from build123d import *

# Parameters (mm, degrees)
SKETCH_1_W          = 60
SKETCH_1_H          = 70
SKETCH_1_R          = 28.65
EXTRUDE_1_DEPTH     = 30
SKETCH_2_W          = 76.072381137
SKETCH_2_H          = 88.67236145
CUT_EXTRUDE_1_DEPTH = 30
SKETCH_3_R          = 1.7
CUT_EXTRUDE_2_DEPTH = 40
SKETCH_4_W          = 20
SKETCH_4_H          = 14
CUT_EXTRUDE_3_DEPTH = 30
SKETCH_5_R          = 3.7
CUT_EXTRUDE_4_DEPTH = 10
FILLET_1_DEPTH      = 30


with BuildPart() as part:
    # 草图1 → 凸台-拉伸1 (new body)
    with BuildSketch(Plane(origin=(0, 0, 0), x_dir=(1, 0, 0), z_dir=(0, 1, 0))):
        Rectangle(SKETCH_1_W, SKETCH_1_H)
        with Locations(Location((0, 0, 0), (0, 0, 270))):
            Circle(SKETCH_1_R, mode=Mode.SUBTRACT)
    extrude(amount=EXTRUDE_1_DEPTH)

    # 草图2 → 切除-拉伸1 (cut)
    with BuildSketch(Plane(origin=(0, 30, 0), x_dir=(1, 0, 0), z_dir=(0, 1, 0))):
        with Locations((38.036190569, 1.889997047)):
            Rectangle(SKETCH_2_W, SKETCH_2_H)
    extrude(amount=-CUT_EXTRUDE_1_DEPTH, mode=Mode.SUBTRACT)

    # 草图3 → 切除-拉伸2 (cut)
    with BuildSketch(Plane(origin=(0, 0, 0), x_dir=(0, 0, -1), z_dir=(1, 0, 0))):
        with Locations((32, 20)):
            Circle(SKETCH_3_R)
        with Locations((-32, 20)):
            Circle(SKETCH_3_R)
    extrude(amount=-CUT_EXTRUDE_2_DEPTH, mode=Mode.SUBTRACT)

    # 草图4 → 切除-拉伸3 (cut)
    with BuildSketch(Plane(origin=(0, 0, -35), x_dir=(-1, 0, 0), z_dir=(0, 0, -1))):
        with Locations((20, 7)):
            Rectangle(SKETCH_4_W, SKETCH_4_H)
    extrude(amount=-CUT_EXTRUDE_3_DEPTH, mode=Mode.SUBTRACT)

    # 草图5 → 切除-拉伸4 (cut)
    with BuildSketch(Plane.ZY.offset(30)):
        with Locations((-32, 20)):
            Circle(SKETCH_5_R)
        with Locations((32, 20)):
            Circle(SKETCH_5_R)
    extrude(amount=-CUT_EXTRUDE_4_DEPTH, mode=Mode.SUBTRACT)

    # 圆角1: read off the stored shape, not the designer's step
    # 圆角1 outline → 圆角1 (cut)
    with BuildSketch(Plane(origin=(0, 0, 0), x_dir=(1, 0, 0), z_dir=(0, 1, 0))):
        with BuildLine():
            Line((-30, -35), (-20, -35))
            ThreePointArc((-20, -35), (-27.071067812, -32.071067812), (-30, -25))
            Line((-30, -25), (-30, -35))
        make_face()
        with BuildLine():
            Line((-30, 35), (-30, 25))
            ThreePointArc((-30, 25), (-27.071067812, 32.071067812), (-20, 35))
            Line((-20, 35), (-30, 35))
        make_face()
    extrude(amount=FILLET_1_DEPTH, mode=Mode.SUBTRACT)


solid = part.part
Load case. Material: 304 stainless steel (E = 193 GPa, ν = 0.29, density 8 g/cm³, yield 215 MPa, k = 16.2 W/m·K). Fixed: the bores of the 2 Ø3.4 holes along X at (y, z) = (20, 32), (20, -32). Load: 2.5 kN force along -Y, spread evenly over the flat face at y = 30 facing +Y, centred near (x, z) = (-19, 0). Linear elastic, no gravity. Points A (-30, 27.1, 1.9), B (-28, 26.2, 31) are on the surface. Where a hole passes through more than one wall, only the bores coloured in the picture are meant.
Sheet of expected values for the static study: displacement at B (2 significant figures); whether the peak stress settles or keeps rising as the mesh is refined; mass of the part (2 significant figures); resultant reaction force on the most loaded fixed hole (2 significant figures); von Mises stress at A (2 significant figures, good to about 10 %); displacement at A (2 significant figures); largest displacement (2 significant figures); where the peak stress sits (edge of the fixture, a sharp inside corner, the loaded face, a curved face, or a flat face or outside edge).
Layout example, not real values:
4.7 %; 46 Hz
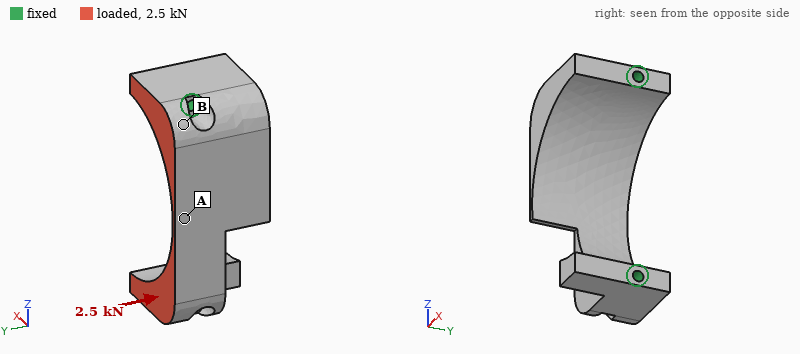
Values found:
1.8 µm; keeps rising; 140 g; 1.3 kN; 14 MPa; 7.2 µm; 8.7 µm; edge of the fixture
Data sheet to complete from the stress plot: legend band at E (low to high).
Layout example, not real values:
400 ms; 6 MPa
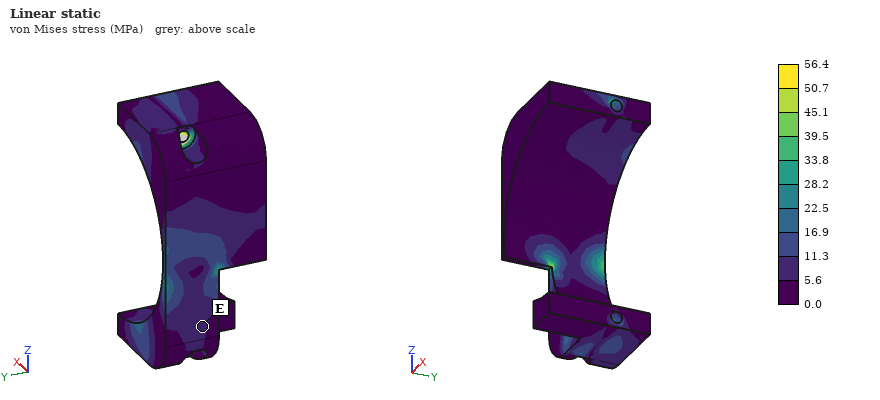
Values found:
5.6 to 11.3 MPa
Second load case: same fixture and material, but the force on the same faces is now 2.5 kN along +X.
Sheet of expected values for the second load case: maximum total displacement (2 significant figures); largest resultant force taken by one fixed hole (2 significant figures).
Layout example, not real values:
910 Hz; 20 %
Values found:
10.0 µm; 1.3 kN
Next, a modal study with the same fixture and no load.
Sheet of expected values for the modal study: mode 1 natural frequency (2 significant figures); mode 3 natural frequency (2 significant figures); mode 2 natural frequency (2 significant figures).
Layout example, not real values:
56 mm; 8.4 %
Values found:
8800 Hz; 12 kHz; 9600 Hz
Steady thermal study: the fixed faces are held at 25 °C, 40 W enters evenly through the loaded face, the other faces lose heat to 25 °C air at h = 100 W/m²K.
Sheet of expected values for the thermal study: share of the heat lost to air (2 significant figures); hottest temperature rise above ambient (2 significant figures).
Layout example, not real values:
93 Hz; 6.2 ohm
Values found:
30 %; 58 K
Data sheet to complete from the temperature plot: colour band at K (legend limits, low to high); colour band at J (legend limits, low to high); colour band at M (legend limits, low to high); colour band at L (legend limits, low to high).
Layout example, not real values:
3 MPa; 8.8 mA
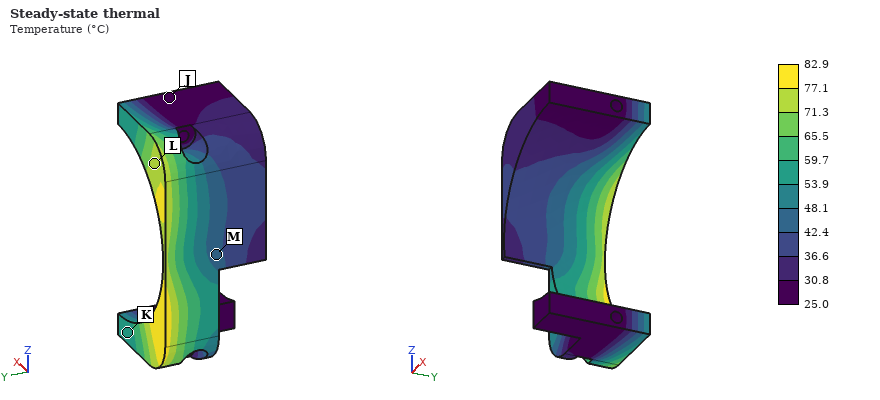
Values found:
53.9 to 59.7 °C; 25.0 to 30.8 °C; 42.4 to 48.1 °C; 71.3 to 77.1 °C
